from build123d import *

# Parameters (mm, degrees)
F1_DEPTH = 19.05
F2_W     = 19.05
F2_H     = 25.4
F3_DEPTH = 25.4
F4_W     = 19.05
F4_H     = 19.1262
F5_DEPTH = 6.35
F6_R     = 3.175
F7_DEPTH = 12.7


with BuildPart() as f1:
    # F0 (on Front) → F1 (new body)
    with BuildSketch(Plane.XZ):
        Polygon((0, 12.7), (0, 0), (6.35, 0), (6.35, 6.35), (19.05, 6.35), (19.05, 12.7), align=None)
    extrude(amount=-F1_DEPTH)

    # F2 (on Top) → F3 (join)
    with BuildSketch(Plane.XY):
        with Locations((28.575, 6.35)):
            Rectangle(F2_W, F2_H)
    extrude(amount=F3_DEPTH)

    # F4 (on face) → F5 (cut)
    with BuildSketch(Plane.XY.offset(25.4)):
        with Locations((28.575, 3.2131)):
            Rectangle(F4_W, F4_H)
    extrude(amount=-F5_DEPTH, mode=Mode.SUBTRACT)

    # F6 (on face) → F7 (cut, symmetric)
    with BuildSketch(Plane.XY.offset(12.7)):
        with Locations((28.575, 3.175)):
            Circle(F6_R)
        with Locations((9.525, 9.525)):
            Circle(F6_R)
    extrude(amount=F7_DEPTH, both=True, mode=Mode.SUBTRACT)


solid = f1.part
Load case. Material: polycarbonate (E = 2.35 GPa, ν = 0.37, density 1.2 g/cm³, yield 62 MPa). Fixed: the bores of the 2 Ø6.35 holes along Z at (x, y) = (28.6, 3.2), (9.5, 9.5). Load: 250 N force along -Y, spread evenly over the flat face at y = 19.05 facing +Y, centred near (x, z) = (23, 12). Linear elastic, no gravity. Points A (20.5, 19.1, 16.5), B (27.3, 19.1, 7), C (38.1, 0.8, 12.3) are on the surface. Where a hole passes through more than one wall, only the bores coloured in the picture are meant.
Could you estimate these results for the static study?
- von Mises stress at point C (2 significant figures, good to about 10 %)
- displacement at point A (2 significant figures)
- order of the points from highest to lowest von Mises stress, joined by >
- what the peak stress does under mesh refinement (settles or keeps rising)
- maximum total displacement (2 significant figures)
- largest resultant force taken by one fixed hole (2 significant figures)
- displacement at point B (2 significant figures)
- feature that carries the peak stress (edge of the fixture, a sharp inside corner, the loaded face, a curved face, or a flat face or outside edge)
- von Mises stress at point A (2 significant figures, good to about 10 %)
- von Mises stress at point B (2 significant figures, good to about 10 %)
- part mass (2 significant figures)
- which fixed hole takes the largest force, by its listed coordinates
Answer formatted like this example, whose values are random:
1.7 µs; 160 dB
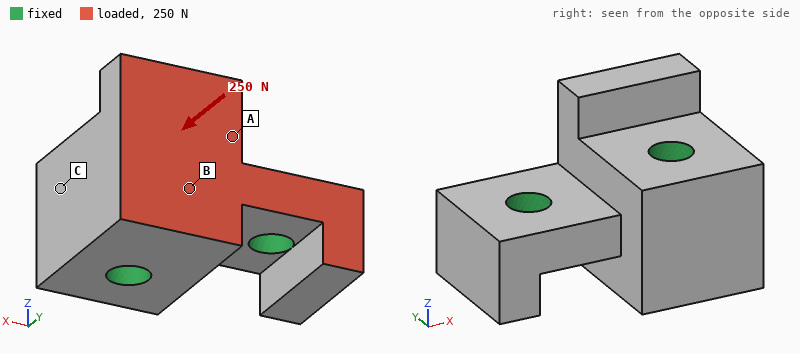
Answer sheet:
0.26 MPa; 6.9 µm; A > B > C; keeps rising; 18 µm; 180 N; 3.4 µm; edge of the fixture; 1.3 MPa; 0.57 MPa; 15 g; (28.6, 3.2)
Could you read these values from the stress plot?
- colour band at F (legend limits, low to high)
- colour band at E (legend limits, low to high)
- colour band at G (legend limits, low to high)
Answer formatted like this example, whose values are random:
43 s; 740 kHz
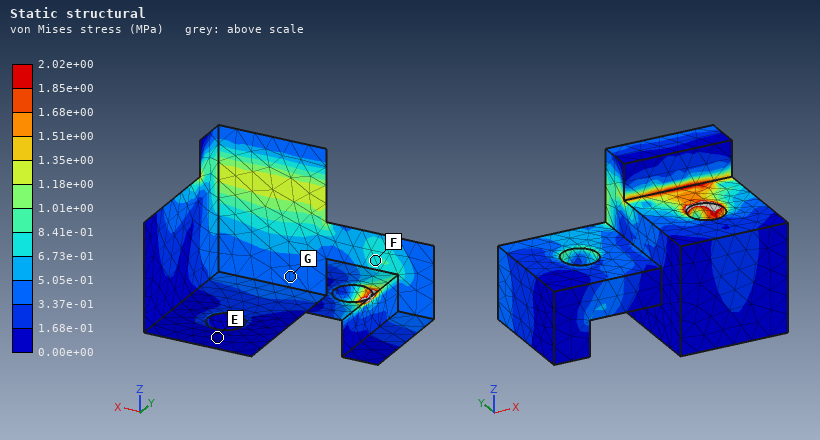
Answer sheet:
6.73e-01 to 8.41e-01 MPa; 0.00e+00 to 1.68e-01 MPa; 3.37e-01 to 5.05e-01 MPa
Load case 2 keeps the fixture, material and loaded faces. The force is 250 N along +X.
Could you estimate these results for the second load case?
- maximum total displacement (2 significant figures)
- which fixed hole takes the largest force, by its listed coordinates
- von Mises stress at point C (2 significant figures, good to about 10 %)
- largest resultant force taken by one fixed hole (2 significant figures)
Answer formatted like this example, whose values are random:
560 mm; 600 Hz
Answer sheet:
31 µm; (9.5, 9.5); 0.52 MPa; 170 N
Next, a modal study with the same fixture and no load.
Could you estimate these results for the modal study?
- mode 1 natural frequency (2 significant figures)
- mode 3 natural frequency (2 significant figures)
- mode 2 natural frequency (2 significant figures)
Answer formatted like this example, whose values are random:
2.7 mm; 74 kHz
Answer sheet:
8100 Hz; 8700 Hz; 8200 Hz
